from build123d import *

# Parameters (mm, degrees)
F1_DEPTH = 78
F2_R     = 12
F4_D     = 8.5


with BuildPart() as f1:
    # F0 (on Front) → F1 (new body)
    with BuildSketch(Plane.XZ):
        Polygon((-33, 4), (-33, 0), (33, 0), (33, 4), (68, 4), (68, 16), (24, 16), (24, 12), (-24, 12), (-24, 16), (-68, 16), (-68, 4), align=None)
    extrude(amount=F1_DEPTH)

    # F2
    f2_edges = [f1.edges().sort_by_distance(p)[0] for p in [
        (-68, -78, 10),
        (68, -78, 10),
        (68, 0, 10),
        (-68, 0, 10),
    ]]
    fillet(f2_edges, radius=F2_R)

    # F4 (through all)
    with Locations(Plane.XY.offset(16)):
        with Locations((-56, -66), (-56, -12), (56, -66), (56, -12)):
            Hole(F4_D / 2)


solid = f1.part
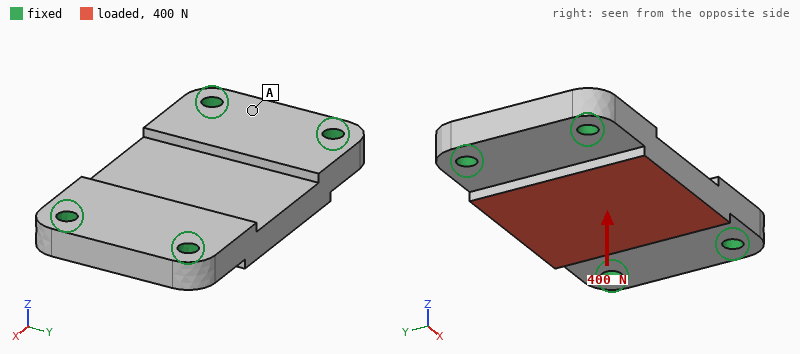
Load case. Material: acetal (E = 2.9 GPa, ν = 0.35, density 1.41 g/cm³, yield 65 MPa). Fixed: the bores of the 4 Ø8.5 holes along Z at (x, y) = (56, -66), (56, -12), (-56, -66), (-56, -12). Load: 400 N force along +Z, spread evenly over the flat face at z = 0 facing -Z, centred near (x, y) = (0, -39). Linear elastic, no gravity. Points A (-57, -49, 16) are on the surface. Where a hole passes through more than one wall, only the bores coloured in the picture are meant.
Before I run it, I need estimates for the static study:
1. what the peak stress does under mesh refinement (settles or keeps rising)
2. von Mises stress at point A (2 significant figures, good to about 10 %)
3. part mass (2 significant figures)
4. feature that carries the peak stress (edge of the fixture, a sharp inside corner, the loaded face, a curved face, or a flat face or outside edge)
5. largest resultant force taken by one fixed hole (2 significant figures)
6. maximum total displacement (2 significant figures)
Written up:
keeps rising
0.66 MPa
180 g
edge of the fixture
170 N
71 µm
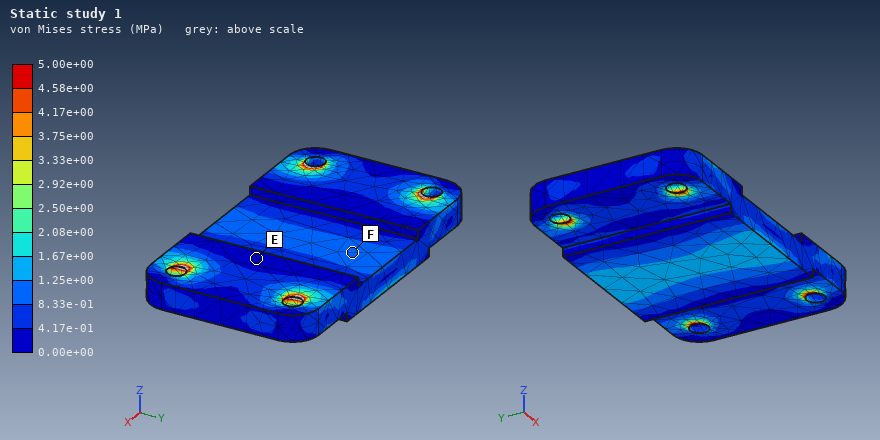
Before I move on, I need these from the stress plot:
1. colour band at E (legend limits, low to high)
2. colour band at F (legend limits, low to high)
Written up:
0.00e+00 to 4.17e-01 MPa
8.33e-01 to 1.25e+00 MPa
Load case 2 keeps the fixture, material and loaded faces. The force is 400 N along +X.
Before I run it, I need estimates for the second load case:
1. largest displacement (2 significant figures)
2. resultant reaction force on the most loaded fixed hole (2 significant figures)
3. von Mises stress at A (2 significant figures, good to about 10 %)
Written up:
5.1 µm
100 N
0.12 MPa
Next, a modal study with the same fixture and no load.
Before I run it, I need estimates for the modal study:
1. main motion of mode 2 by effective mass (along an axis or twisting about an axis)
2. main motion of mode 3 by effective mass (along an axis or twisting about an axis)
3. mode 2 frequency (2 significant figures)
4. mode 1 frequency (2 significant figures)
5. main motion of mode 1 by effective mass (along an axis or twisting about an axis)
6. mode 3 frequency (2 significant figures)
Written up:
twisting about X
twisting about Y
1900 Hz
1300 Hz
along Z
3100 Hz
